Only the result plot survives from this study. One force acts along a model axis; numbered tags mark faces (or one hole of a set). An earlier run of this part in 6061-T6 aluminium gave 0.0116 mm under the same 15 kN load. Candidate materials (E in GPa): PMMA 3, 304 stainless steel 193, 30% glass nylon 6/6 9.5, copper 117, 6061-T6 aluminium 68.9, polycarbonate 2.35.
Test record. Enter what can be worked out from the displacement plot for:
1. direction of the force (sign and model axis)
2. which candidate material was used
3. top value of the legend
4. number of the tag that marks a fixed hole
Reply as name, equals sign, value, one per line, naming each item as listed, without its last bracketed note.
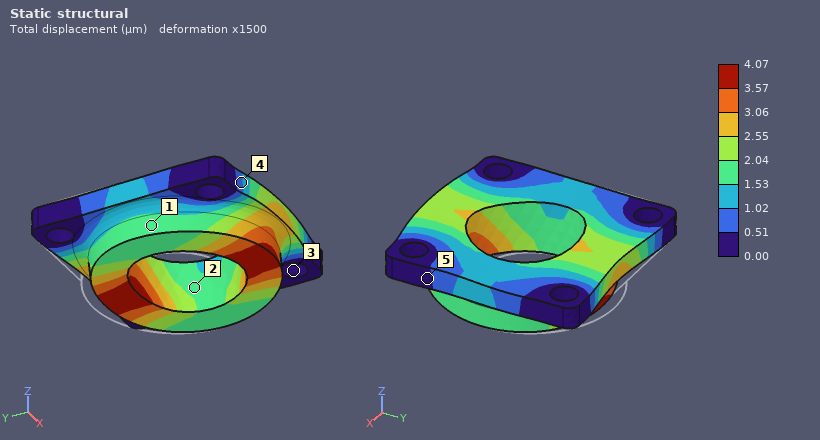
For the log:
direction of the force = -Y
which candidate material was used = 304 stainless steel
top value of the legend = 4.07 µm
number of the tag that marks a fixed hole = 3
